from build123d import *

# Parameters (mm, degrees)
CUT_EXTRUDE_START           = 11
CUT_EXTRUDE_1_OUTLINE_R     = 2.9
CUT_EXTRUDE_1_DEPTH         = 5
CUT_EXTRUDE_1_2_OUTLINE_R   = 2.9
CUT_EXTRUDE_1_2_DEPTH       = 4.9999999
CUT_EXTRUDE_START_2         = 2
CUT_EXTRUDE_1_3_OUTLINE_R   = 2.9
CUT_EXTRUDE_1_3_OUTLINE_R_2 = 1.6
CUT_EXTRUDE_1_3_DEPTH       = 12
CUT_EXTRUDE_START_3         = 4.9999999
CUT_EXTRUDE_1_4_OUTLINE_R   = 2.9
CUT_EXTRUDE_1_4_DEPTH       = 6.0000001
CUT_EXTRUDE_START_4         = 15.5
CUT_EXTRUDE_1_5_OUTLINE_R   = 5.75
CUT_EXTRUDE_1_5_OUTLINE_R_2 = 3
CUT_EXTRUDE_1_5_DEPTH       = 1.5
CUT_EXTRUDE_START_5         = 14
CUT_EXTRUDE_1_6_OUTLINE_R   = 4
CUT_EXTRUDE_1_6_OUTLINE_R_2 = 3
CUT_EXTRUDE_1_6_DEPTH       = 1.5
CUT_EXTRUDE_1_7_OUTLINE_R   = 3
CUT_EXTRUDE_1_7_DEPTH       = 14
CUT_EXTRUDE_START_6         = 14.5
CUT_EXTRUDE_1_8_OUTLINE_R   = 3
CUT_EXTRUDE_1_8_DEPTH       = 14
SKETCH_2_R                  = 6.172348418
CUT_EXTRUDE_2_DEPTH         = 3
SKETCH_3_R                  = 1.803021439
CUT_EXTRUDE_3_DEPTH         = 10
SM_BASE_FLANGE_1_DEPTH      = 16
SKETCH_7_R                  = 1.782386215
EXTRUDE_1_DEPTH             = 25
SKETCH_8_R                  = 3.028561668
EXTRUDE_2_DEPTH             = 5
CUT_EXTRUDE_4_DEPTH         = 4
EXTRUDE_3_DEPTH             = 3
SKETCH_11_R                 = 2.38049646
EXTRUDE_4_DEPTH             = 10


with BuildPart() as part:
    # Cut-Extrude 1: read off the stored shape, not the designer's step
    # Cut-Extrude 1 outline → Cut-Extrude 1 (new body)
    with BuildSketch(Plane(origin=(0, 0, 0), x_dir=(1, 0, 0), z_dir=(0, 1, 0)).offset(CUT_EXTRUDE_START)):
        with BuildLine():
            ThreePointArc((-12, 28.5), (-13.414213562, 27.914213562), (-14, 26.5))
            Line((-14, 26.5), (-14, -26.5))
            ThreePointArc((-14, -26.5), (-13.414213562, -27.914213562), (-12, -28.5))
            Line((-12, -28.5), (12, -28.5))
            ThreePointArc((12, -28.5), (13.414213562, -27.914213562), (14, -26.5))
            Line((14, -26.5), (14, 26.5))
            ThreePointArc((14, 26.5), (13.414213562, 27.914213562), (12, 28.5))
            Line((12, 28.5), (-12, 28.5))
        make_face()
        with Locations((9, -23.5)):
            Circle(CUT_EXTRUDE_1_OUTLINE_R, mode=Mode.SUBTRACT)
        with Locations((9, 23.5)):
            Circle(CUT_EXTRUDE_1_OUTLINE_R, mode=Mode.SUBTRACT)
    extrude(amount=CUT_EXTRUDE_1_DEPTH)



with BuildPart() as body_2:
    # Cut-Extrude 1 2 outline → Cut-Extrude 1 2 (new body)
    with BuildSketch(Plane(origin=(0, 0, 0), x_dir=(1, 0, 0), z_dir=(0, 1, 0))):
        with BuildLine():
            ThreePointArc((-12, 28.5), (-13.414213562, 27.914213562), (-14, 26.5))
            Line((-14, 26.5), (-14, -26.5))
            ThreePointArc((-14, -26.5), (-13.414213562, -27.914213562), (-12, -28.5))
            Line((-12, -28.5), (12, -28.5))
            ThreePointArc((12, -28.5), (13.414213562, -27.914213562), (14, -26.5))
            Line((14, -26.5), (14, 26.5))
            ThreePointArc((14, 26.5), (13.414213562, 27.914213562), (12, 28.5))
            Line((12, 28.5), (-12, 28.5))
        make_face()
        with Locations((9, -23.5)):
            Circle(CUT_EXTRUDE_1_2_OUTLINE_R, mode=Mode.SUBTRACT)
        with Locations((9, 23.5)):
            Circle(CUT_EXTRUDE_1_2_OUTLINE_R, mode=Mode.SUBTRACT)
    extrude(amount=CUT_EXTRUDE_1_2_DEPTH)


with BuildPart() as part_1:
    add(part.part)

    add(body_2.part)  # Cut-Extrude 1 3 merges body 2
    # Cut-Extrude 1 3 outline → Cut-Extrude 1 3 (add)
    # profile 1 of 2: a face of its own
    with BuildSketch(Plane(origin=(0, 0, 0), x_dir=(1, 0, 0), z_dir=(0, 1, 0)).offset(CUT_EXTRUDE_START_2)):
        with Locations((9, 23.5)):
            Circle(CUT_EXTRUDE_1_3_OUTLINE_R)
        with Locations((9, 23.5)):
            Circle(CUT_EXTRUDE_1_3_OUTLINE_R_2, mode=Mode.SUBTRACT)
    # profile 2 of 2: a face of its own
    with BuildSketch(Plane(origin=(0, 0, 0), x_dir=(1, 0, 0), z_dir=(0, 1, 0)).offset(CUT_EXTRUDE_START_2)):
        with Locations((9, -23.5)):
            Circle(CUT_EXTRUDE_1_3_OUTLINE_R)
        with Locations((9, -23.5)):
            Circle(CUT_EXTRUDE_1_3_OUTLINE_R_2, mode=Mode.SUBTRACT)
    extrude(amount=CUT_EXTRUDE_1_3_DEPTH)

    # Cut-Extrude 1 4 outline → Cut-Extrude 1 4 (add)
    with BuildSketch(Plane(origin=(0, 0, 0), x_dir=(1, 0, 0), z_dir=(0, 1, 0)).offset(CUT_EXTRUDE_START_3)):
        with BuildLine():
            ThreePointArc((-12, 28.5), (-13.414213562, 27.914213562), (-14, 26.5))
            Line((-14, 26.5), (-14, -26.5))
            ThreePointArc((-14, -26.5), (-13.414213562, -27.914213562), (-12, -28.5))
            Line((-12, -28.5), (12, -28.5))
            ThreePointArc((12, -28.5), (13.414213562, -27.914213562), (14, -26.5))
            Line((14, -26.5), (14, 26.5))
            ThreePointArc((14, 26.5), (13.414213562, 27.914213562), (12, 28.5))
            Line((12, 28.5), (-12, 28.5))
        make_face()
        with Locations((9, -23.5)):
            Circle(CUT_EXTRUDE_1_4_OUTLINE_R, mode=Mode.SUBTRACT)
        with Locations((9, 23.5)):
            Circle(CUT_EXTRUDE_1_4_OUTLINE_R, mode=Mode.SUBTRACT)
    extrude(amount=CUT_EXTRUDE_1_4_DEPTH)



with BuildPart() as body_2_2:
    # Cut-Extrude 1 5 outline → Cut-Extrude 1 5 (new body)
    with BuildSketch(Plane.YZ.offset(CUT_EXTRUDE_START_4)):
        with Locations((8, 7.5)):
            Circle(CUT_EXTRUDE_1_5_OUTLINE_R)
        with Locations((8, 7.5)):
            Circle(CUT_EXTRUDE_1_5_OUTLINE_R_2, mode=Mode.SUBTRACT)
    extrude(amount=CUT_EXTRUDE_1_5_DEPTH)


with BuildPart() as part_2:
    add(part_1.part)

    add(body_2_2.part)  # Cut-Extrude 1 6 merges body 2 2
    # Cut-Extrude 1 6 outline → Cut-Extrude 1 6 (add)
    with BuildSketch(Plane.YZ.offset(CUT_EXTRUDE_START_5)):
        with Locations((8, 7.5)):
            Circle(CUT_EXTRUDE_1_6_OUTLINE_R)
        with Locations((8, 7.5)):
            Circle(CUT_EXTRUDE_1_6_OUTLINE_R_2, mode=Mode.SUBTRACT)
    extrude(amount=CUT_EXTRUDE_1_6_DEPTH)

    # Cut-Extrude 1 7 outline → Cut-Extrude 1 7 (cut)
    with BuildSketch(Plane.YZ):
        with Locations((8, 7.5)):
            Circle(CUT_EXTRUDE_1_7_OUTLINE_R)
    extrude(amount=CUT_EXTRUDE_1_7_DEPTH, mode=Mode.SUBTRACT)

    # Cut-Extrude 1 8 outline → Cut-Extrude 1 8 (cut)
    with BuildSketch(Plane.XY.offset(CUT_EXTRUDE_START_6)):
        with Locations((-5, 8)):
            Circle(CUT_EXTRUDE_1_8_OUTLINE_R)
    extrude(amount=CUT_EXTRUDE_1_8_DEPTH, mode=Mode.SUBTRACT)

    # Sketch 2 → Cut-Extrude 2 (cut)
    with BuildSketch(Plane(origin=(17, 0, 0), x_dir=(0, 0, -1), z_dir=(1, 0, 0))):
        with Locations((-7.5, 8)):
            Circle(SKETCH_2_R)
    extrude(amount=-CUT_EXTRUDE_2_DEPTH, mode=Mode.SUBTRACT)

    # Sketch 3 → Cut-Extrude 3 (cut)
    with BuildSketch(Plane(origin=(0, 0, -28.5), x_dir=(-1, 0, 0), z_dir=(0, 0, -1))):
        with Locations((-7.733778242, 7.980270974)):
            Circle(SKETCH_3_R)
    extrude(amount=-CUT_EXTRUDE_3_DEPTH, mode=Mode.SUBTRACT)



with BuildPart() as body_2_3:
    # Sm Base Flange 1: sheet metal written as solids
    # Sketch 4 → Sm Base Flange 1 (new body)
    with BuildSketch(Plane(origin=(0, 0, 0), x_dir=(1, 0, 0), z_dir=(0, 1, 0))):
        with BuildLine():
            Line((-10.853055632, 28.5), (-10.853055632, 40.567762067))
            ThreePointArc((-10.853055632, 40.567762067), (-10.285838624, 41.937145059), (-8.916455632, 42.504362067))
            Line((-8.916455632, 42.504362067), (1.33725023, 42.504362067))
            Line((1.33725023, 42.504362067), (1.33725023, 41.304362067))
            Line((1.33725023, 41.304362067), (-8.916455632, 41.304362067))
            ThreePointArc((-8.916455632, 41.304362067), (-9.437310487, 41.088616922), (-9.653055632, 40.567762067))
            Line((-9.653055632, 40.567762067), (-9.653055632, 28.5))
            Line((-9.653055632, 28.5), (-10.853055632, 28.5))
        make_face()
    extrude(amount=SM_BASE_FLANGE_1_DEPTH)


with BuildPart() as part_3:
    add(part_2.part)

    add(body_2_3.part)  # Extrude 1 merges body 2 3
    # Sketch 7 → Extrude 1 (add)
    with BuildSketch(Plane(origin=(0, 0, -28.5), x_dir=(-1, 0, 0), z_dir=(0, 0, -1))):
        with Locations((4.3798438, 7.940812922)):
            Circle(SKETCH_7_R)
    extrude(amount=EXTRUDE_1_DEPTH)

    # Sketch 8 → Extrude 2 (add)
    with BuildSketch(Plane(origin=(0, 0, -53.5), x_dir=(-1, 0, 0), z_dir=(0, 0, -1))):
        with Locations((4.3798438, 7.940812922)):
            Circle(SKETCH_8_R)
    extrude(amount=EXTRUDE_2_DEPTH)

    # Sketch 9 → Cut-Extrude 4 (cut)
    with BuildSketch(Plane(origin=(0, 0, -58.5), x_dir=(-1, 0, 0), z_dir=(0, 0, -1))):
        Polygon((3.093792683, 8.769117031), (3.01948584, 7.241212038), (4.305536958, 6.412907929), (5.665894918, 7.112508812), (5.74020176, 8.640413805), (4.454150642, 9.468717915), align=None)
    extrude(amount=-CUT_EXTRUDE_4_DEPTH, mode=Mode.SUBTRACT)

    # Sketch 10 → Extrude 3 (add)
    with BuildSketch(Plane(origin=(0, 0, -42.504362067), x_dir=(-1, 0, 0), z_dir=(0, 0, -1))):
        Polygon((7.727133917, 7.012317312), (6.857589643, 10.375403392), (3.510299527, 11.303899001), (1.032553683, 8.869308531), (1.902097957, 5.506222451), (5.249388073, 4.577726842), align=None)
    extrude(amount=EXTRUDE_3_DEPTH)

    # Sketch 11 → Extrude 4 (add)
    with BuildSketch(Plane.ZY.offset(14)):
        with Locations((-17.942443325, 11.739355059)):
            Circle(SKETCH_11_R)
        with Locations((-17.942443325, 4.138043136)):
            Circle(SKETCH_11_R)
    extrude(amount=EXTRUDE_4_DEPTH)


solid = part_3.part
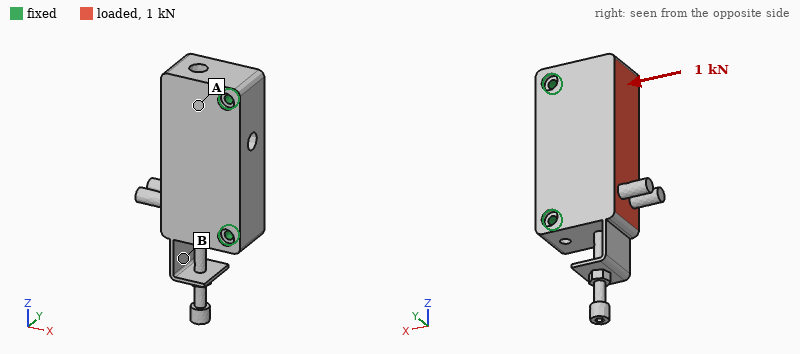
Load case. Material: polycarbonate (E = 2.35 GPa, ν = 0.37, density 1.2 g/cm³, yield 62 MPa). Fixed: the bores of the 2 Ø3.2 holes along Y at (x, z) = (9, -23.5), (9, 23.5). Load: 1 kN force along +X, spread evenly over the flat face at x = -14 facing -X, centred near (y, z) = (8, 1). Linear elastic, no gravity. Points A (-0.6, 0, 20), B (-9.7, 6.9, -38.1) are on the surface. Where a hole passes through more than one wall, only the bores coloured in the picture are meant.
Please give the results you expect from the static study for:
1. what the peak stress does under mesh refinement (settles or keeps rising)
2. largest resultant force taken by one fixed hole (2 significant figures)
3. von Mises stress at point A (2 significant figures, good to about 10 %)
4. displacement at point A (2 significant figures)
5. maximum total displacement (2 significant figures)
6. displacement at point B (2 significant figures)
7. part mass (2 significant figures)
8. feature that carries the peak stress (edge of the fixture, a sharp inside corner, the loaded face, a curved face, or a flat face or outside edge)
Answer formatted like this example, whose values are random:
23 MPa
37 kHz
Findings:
keeps rising
550 N
2.3 MPa
18 µm
38 µm
6.8 µm
31 g
edge of the fixture
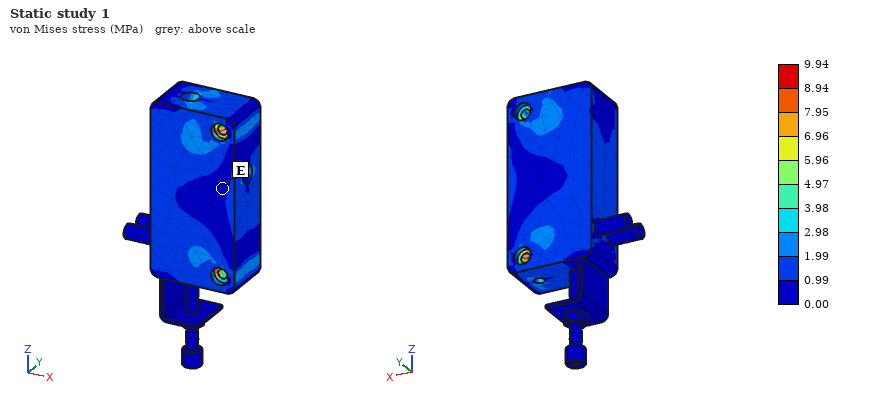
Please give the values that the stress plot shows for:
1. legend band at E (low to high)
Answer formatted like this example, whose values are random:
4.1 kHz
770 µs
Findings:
0.00 to 0.99 MPa
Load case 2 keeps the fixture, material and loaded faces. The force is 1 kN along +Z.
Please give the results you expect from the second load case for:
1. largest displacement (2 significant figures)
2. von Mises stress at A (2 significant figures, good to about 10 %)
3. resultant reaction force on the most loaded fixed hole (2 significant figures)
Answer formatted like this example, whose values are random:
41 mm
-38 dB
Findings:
0.10 mm
2.1 MPa
690 N
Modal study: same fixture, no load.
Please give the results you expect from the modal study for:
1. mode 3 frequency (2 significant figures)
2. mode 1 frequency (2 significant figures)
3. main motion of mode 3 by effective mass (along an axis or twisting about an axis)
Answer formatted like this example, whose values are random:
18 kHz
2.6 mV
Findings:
2400 Hz
1200 Hz
along Y
